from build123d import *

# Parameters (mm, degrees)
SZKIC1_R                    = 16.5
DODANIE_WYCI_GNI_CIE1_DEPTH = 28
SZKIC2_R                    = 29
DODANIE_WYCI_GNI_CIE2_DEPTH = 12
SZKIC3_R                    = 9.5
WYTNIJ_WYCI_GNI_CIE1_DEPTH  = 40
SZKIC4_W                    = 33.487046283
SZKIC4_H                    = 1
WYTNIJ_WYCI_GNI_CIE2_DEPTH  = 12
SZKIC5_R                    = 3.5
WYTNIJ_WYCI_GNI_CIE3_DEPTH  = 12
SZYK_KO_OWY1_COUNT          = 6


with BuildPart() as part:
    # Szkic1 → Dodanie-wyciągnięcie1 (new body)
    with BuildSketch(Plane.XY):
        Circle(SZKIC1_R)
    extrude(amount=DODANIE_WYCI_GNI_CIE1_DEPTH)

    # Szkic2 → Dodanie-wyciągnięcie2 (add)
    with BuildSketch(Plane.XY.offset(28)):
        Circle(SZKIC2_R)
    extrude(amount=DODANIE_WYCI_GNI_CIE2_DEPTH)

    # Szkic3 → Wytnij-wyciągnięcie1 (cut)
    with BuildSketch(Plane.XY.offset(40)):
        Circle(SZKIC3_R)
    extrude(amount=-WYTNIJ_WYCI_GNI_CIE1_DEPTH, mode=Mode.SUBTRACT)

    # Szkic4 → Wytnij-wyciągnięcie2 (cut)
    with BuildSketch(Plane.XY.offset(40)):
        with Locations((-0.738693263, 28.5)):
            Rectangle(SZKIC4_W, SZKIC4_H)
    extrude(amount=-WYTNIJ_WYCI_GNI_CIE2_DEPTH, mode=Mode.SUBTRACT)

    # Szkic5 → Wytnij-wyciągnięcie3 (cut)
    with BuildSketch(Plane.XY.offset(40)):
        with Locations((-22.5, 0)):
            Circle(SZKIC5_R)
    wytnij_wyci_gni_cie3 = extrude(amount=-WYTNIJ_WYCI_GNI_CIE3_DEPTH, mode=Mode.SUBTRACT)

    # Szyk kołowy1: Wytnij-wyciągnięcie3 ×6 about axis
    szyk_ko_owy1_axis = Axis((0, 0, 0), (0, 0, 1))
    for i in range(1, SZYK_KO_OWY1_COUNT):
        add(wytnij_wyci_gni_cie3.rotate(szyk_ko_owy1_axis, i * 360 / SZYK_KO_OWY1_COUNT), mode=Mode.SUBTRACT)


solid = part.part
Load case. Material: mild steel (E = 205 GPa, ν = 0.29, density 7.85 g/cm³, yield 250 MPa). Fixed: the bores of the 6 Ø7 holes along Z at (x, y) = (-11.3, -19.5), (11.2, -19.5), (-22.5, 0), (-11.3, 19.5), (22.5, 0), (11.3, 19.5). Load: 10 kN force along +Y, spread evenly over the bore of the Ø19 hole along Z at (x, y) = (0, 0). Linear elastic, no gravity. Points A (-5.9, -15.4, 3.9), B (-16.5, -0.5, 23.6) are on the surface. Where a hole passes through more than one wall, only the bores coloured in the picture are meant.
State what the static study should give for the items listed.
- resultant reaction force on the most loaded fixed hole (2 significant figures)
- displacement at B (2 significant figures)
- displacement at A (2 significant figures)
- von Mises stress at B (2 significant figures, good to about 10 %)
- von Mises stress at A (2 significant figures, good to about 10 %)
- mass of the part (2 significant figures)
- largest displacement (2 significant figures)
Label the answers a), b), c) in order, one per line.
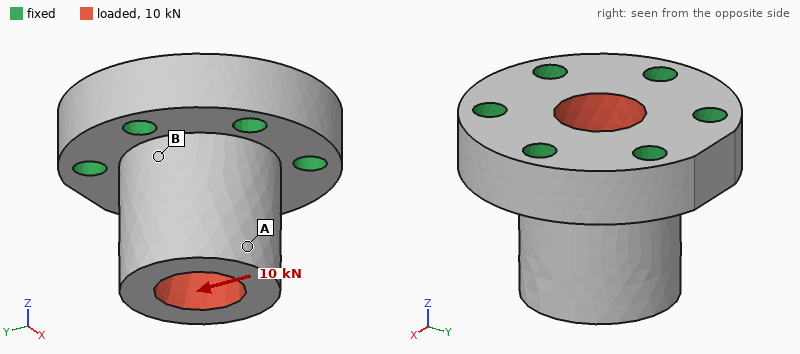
a) 2.9 kN
b) 2.0 µm
c) 7.9 µm
d) 20 MPa
e) 7.2 MPa
f) 330 g
g) 8.9 µm
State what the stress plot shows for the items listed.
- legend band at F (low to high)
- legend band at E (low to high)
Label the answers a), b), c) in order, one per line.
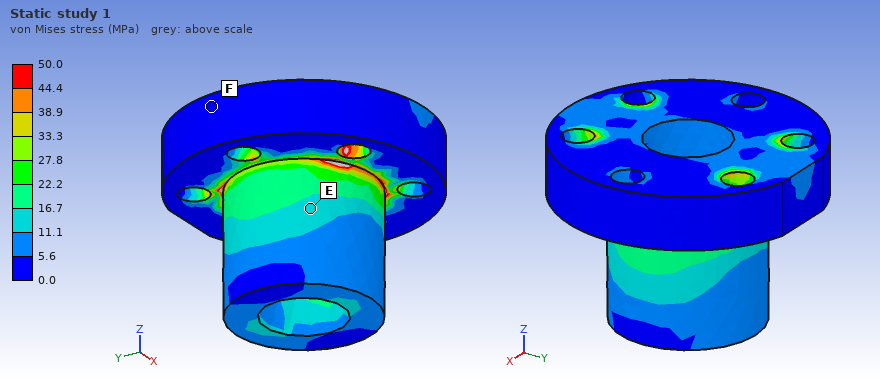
a) 0.0 to 5.6 MPa
b) 11.1 to 16.7 MPa
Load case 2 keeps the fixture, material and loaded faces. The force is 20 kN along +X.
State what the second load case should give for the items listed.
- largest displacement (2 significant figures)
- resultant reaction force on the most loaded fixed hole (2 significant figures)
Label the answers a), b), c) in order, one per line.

a) 18 µm
b) 6.5 kN
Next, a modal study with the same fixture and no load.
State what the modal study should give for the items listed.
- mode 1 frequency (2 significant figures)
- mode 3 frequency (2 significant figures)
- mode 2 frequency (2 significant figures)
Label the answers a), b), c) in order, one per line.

a) 15 kHz
b) 25 kHz
c) 15 kHz
